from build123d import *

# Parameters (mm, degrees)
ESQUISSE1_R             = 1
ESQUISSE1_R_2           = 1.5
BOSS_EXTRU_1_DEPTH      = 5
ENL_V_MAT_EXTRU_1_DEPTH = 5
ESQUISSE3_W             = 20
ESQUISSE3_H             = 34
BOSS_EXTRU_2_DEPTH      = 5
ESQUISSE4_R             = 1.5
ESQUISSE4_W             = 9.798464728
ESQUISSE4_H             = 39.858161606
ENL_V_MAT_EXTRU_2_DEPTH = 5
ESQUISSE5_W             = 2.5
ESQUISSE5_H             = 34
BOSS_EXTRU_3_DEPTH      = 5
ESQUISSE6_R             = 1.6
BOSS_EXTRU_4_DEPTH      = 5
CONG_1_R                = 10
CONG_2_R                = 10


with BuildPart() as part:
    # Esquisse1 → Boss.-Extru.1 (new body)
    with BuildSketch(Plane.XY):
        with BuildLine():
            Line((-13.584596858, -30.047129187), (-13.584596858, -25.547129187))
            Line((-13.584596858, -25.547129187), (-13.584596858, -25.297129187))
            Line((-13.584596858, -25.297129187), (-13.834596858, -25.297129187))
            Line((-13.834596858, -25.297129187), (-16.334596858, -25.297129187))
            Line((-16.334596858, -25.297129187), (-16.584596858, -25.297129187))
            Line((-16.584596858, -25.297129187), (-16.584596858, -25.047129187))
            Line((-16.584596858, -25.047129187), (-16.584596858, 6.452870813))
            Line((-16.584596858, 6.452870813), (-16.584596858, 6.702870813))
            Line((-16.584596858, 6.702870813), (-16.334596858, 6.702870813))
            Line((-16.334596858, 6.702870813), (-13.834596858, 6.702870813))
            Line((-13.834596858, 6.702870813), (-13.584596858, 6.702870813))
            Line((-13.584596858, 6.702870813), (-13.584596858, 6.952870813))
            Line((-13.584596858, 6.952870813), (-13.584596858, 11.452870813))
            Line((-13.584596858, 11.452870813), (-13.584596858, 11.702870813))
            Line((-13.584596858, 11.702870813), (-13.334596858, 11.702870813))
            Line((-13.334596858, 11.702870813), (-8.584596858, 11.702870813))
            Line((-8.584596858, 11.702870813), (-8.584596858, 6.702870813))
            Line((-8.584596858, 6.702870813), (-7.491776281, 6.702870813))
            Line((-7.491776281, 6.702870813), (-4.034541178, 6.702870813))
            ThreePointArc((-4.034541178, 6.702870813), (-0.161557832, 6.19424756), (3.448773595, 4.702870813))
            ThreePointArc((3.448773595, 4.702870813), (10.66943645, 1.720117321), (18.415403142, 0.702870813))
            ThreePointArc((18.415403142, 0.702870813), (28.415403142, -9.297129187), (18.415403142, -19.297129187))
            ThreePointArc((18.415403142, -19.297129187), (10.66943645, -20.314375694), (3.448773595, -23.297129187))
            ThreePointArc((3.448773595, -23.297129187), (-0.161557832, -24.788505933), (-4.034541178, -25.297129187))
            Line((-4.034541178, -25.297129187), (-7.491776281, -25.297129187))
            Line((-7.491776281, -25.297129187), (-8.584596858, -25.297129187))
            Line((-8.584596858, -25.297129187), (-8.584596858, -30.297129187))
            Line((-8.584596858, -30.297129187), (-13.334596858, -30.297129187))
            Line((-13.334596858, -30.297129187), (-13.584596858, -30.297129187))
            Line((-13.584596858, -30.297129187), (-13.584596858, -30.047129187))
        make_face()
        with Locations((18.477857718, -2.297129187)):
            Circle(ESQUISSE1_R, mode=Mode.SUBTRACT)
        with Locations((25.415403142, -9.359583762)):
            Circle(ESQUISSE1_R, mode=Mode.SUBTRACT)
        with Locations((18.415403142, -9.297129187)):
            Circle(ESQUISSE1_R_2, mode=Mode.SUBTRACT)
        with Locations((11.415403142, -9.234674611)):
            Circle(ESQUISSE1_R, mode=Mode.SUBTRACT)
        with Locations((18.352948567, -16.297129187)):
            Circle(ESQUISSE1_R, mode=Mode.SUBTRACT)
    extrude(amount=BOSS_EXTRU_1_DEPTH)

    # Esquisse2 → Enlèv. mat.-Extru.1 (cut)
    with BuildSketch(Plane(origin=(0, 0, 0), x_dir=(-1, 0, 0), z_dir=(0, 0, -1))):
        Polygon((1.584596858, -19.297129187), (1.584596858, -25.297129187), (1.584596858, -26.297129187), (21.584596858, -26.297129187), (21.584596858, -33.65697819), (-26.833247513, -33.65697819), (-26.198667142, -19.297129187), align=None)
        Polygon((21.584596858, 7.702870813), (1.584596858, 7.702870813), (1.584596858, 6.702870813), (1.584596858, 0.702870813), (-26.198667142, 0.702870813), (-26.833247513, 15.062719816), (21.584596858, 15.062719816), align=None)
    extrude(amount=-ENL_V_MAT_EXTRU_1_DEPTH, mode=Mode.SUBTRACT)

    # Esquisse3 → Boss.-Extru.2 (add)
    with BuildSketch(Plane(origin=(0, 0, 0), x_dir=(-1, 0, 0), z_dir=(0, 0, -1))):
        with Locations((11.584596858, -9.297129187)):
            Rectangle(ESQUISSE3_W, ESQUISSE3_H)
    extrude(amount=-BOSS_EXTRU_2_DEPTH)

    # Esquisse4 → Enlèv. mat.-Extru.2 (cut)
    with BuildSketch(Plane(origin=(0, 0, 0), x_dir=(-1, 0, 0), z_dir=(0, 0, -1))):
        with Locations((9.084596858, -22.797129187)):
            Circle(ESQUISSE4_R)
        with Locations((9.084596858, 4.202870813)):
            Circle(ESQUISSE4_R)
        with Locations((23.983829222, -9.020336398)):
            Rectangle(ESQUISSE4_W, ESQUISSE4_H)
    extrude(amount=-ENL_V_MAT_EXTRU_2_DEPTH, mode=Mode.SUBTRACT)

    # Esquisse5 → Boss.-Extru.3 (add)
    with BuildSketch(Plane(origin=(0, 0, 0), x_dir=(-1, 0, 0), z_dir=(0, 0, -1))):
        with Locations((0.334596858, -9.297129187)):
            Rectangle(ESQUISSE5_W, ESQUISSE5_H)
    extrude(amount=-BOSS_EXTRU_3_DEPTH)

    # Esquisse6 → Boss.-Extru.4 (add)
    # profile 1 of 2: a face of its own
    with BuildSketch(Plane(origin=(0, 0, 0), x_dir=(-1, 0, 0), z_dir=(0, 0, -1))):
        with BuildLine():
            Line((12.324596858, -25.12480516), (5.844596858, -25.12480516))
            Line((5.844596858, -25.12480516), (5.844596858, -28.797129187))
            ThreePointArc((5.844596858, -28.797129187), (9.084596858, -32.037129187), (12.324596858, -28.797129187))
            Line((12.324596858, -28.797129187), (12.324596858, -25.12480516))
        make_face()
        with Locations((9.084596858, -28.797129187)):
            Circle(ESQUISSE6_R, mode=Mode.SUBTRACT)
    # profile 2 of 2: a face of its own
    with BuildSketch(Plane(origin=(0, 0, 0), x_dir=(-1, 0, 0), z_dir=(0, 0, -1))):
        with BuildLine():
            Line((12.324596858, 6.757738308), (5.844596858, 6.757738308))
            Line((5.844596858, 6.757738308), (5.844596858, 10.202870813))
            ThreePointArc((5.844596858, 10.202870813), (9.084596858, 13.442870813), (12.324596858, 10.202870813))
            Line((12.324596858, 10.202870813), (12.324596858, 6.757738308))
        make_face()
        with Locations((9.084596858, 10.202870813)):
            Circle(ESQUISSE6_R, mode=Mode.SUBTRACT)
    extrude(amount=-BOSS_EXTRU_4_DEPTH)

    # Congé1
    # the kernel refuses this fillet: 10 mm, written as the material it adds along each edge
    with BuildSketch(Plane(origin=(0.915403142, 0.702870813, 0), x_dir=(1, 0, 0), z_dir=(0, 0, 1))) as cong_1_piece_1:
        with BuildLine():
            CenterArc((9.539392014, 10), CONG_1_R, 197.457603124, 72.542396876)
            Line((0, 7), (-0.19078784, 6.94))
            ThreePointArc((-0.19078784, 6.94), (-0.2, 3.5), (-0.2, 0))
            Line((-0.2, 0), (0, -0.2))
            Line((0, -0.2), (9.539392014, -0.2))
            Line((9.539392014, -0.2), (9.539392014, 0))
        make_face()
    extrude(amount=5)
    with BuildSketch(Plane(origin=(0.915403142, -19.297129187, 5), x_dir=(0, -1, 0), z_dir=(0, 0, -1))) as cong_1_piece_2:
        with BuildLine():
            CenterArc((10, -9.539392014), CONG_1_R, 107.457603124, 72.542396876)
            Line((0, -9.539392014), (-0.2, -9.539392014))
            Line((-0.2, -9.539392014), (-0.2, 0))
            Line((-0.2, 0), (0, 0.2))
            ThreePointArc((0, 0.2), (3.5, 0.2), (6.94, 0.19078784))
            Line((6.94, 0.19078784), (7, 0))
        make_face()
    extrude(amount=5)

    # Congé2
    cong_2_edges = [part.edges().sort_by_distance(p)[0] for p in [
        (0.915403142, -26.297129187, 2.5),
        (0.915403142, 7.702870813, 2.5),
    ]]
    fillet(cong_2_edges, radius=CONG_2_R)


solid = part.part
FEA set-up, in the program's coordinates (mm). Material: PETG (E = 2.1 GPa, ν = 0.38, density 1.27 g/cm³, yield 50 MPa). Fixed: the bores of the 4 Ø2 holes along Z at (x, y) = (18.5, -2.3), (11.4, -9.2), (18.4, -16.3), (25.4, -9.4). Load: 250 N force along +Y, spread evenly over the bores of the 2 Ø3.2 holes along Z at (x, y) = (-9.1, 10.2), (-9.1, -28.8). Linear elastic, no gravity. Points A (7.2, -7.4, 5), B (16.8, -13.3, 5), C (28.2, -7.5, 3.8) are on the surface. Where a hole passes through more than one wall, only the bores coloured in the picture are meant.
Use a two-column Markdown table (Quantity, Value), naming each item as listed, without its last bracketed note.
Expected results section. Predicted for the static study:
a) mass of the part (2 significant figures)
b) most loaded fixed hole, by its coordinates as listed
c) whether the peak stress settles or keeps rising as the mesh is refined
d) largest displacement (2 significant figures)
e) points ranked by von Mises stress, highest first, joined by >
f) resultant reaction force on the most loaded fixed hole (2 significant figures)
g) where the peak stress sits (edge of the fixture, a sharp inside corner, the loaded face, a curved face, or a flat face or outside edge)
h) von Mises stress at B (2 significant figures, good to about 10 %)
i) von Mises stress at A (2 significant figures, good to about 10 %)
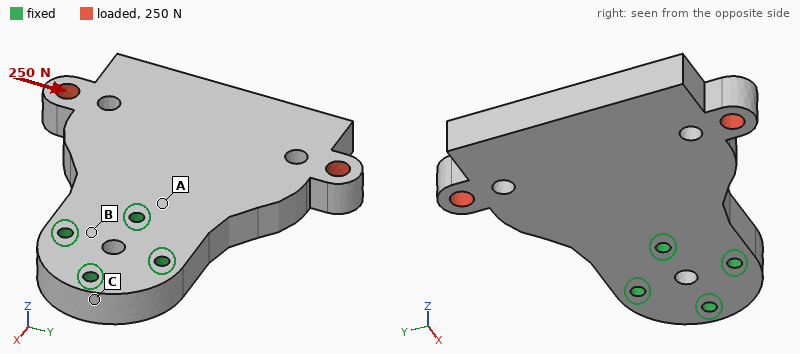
| Quantity | Value |
|---|---|
| mass of the part | 7.8 g |
| most loaded fixed hole, by its coordinates as listed | (11.4, -9.2) |
| whether the peak stress settles or keeps rising as the mesh is refined | keeps rising |
| largest displacement | 0.44 mm |
| points ranked by von Mises stress, highest first, joined by > | A > B > C |
| resultant reaction force on the most loaded fixed hole | 330 N |
| where the peak stress sits | edge of the fixture |
| von Mises stress at B | 3.3 MPa |
| von Mises stress at A | 7.2 MPa |
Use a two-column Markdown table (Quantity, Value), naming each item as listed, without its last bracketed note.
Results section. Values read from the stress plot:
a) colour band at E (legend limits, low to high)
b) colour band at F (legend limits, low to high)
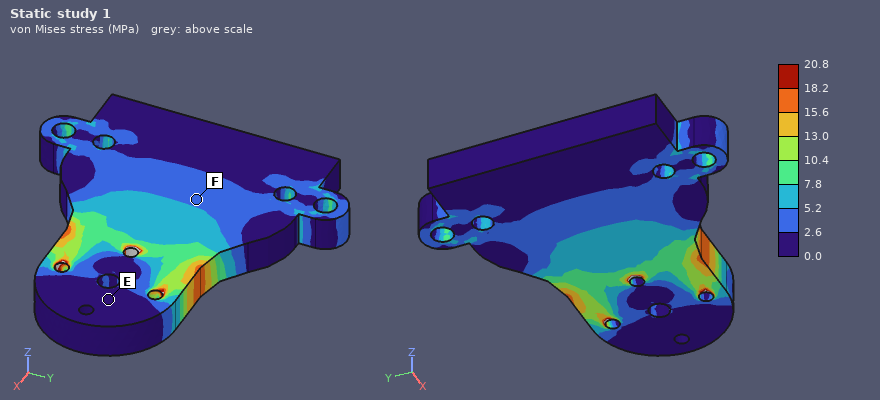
| Quantity | Value |
|---|---|
| colour band at E | 0.0 to 2.6 MPa |
| colour band at F | 2.6 to 5.2 MPa |
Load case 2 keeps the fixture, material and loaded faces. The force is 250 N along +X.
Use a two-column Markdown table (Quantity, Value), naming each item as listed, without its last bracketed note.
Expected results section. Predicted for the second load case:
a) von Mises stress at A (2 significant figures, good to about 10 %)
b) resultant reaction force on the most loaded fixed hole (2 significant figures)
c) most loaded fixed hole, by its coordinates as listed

| Quantity | Value |
|---|---|
| von Mises stress at A | 2.4 MPa |
| resultant reaction force on the most loaded fixed hole | 120 N |
| most loaded fixed hole, by its coordinates as listed | (11.4, -9.2) |
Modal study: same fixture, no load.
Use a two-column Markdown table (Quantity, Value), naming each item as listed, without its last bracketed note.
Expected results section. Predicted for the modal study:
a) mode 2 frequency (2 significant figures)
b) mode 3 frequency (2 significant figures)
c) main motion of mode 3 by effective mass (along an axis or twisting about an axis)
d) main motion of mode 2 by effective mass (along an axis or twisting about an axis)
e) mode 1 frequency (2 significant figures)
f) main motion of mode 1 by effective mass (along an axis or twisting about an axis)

| Quantity | Value |
|---|---|
| mode 2 frequency | 1300 Hz |
| mode 3 frequency | 2000 Hz |
| main motion of mode 3 by effective mass | along Y |
| main motion of mode 2 by effective mass | twisting about X |
| mode 1 frequency | 810 Hz |
| main motion of mode 1 by effective mass | along Z |
